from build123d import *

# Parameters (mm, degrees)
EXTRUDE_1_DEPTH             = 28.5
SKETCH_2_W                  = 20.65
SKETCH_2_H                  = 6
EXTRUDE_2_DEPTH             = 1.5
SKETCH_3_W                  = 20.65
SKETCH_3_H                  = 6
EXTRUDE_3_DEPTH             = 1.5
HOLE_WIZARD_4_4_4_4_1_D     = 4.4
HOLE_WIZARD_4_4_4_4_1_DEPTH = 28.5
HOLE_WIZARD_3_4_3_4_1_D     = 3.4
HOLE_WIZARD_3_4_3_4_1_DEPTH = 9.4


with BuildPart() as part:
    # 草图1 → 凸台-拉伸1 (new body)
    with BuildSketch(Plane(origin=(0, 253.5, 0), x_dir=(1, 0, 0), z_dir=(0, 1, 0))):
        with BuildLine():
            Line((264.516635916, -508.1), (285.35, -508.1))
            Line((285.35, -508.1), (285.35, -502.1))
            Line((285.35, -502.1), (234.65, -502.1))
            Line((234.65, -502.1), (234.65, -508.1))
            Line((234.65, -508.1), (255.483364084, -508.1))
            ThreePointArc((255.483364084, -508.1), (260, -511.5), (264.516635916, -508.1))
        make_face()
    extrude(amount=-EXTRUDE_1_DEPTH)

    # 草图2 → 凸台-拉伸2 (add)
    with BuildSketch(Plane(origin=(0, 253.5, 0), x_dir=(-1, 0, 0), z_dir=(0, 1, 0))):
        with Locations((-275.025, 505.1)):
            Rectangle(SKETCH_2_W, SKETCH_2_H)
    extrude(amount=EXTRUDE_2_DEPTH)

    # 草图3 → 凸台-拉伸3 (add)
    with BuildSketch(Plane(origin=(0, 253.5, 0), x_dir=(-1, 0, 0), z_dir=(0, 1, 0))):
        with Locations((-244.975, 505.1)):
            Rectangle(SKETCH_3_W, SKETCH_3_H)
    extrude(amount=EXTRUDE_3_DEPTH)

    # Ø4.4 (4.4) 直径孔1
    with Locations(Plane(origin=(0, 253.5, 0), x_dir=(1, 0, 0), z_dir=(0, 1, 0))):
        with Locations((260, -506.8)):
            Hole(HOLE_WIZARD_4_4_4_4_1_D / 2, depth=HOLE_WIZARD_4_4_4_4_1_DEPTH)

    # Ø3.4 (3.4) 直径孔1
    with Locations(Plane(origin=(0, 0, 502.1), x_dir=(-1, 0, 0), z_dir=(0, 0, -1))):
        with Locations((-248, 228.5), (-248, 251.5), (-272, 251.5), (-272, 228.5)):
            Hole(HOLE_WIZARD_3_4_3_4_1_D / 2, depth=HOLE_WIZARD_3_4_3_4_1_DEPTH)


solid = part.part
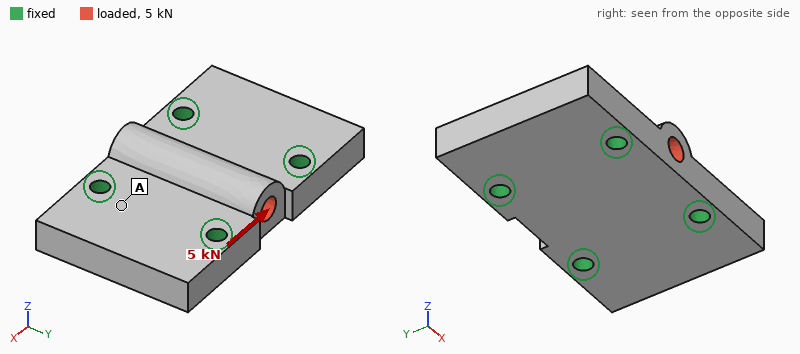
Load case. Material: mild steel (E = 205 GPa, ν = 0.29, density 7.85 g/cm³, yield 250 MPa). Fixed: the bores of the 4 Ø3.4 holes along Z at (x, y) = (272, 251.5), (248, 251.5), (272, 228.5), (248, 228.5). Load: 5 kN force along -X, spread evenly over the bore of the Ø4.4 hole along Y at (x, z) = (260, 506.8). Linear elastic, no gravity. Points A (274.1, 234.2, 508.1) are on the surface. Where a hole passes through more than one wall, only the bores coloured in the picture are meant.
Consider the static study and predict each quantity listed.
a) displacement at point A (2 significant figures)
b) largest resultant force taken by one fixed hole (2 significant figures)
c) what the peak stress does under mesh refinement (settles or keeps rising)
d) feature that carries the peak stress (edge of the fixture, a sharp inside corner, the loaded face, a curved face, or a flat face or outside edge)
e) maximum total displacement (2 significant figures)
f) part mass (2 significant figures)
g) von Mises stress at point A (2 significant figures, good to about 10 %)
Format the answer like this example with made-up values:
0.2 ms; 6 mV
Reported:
0.50 µm; 1.3 kN; keeps rising; a sharp inside corner; 1.8 µm; 71 g; 7.7 MPa
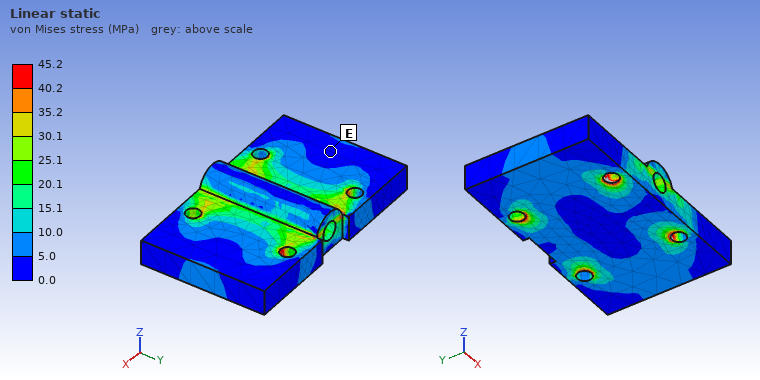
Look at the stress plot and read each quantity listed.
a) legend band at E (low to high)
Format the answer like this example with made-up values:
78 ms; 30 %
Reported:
0.0 to 5.0 MPa
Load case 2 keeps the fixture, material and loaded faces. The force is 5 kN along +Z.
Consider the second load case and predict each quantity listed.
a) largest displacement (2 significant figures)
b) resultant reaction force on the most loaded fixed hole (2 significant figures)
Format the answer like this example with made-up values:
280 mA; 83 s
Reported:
6.8 µm; 1.3 kN
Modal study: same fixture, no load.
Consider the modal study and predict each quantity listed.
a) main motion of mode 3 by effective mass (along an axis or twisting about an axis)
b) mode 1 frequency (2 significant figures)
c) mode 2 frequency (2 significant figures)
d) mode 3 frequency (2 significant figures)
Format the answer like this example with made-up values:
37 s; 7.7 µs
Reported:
along Z; 21 kHz; 21 kHz; 33 kHz
